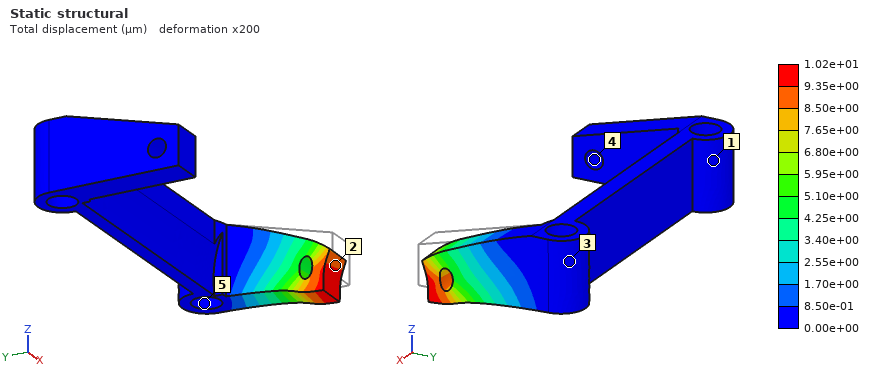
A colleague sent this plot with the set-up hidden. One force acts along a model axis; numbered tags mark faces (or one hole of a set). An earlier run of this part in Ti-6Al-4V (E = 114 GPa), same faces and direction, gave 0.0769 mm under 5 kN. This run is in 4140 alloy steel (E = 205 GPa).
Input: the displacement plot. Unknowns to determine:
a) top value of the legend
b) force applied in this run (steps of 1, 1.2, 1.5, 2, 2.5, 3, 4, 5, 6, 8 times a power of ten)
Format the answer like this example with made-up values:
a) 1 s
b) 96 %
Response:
a) 1.02e+01 µm
b) 1.2 kN
